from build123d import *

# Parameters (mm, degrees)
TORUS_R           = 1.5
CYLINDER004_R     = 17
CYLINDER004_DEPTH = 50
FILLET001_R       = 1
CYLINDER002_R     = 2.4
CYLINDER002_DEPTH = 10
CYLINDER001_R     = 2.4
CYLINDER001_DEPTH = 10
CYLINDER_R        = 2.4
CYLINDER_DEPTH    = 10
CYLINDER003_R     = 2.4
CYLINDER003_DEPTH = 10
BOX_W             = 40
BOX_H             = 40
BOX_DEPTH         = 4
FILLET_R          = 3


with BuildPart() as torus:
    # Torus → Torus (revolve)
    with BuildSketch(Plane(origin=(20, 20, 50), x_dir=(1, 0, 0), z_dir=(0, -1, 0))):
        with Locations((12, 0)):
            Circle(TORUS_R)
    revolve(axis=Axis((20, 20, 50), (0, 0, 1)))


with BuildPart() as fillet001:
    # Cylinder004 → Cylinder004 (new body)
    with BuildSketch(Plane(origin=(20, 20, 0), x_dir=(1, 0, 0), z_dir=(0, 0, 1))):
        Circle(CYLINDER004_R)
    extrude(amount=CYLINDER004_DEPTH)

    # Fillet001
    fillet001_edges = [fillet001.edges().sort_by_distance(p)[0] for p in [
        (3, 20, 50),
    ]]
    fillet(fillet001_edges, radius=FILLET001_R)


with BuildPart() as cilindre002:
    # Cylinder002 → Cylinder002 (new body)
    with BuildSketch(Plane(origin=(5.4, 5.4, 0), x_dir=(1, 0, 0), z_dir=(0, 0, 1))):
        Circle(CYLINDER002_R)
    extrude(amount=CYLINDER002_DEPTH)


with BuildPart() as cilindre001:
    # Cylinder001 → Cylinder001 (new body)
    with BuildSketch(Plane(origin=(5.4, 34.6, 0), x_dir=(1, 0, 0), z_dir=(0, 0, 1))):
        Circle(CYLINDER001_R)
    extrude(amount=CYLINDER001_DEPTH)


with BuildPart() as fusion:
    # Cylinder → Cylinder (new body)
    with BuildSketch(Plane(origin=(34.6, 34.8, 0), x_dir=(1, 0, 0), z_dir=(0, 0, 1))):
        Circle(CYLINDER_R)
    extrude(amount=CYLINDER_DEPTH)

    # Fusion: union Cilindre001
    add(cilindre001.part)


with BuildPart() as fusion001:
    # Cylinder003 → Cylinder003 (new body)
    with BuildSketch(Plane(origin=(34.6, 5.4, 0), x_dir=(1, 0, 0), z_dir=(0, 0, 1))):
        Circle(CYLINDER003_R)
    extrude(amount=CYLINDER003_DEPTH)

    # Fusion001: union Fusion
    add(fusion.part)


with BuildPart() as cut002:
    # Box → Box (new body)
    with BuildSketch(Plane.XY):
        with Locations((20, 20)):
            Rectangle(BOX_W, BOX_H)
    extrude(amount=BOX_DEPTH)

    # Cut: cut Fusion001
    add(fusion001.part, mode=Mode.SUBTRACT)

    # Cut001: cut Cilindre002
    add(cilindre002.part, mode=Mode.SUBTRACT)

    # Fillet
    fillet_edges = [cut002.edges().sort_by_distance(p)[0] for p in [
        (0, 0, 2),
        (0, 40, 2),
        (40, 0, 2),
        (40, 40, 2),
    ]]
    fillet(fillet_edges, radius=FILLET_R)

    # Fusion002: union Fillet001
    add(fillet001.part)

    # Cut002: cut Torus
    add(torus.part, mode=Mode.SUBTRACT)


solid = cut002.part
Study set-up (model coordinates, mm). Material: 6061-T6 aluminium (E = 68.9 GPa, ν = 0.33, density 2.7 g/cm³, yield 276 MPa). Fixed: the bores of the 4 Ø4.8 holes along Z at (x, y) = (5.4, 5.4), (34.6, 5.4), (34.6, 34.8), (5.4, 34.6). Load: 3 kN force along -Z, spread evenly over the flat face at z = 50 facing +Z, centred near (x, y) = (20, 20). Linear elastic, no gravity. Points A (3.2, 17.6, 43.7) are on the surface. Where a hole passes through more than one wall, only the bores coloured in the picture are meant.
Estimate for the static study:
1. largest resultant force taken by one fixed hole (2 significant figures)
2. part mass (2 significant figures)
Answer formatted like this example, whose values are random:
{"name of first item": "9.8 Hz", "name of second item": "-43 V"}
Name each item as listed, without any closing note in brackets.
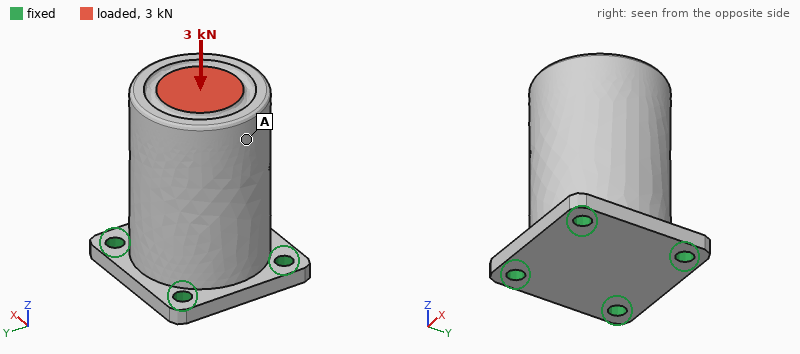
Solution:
{"largest resultant force taken by one fixed hole": "820 N", "part mass": "130 g"}
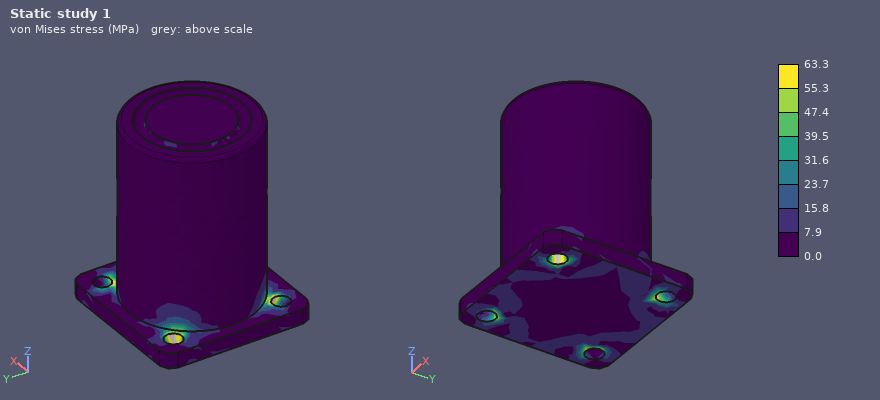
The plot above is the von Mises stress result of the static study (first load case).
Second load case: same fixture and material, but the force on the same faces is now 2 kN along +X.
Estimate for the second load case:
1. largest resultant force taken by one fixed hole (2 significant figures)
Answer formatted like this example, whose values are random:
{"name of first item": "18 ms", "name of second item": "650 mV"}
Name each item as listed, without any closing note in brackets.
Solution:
{"largest resultant force taken by one fixed hole": "2.0 kN"}
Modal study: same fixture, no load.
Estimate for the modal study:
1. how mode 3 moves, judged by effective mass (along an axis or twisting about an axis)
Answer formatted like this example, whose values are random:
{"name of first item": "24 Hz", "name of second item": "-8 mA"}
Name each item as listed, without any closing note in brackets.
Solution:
{"how mode 3 moves, judged by effective mass": "along Z"}
